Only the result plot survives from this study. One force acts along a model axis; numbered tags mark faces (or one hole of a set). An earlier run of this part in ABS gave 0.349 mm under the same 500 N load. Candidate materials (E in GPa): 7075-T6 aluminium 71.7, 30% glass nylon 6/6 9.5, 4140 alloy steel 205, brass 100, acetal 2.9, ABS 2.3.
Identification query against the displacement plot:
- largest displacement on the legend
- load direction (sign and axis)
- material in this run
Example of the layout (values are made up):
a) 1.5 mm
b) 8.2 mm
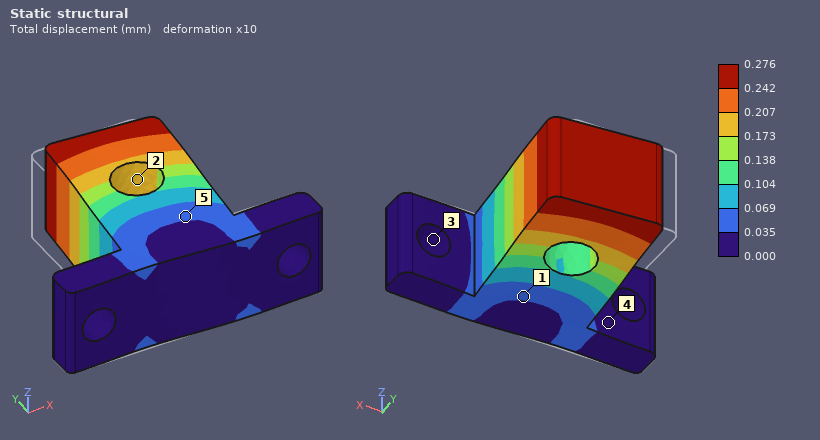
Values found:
a) 0.276 mm
b) +X
c) acetal
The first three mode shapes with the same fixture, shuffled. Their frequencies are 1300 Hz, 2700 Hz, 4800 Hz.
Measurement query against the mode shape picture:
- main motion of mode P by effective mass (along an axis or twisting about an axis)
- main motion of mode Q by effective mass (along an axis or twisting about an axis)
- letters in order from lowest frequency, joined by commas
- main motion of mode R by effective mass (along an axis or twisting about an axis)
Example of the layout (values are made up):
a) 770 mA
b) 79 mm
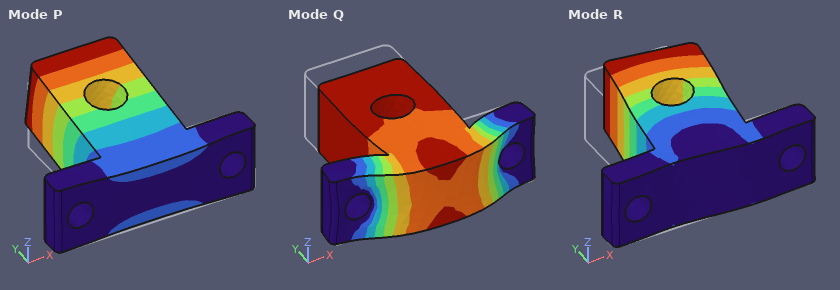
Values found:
a) along Z
b) along Y
c) P, R, Q
d) along X
